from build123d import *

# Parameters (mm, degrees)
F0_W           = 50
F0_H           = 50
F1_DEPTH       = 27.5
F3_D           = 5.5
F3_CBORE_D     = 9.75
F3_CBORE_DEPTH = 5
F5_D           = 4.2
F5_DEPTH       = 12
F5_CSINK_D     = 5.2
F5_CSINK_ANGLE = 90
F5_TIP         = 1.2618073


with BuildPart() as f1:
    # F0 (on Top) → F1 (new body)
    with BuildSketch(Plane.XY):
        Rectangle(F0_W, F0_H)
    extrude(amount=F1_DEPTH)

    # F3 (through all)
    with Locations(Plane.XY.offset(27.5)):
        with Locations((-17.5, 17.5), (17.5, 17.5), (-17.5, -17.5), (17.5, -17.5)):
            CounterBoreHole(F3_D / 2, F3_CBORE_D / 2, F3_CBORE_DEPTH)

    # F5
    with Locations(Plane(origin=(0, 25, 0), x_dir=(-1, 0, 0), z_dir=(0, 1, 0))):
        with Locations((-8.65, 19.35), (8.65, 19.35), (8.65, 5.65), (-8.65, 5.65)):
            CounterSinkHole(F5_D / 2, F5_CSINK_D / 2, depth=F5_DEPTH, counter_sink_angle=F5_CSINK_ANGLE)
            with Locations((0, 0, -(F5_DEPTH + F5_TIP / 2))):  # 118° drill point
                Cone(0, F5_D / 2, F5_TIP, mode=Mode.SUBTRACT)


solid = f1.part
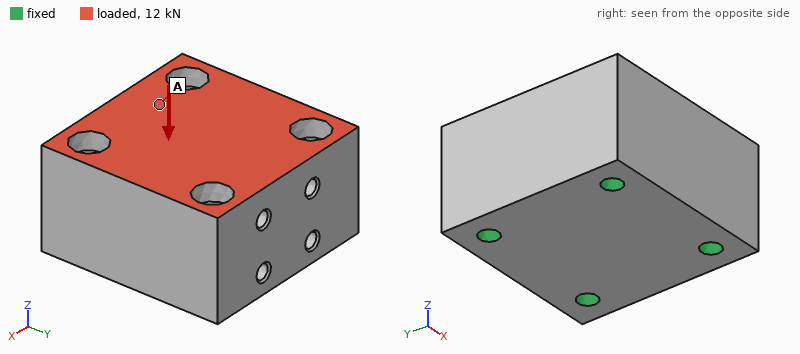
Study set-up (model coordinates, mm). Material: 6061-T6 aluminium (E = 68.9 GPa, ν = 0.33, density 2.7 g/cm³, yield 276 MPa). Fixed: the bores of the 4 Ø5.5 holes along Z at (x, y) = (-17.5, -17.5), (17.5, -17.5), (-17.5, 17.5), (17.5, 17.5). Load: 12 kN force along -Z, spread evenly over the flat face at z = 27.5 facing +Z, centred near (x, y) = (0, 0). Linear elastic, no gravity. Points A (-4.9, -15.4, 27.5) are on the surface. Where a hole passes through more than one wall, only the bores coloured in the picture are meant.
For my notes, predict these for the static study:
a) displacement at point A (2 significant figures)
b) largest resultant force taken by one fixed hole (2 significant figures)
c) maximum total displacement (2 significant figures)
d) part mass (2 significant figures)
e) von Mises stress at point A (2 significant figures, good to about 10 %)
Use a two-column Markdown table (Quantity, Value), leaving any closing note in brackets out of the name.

| Quantity | Value |
|---|---|
| displacement at point A | 2.6 µm |
| largest resultant force taken by one fixed hole | 3.1 kN |
| maximum total displacement | 3.2 µm |
| part mass | 170 g |
| von Mises stress at point A | 4.5 MPa |
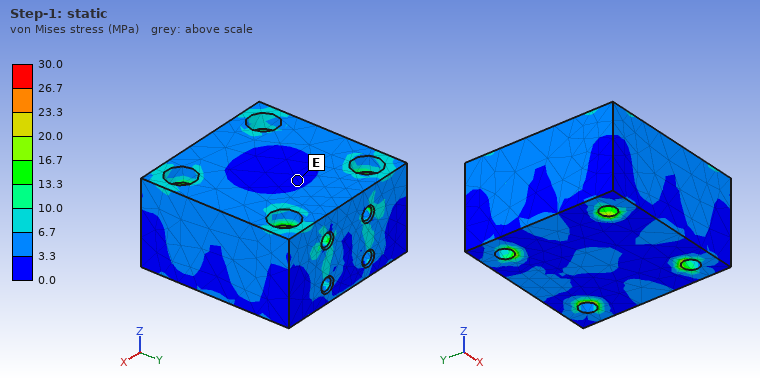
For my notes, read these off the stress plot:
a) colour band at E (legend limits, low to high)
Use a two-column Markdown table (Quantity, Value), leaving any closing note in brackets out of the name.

| Quantity | Value |
|---|---|
| colour band at E | 0.0 to 3.3 MPa |
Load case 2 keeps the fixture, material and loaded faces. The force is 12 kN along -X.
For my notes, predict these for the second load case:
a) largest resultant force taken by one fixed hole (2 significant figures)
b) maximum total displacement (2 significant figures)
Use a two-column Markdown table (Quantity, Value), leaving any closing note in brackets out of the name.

| Quantity | Value |
|---|---|
| largest resultant force taken by one fixed hole | 3.6 kN |
| maximum total displacement | 7.4 µm |
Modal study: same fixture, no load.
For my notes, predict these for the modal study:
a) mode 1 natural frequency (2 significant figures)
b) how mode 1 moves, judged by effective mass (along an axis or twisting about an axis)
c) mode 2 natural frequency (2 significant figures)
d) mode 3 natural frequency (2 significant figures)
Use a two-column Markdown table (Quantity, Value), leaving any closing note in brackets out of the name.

| Quantity | Value |
|---|---|
| mode 1 natural frequency | 30 kHz |
| how mode 1 moves, judged by effective mass | along Z |
| mode 2 natural frequency | 35 kHz |
| mode 3 natural frequency | 36 kHz |
